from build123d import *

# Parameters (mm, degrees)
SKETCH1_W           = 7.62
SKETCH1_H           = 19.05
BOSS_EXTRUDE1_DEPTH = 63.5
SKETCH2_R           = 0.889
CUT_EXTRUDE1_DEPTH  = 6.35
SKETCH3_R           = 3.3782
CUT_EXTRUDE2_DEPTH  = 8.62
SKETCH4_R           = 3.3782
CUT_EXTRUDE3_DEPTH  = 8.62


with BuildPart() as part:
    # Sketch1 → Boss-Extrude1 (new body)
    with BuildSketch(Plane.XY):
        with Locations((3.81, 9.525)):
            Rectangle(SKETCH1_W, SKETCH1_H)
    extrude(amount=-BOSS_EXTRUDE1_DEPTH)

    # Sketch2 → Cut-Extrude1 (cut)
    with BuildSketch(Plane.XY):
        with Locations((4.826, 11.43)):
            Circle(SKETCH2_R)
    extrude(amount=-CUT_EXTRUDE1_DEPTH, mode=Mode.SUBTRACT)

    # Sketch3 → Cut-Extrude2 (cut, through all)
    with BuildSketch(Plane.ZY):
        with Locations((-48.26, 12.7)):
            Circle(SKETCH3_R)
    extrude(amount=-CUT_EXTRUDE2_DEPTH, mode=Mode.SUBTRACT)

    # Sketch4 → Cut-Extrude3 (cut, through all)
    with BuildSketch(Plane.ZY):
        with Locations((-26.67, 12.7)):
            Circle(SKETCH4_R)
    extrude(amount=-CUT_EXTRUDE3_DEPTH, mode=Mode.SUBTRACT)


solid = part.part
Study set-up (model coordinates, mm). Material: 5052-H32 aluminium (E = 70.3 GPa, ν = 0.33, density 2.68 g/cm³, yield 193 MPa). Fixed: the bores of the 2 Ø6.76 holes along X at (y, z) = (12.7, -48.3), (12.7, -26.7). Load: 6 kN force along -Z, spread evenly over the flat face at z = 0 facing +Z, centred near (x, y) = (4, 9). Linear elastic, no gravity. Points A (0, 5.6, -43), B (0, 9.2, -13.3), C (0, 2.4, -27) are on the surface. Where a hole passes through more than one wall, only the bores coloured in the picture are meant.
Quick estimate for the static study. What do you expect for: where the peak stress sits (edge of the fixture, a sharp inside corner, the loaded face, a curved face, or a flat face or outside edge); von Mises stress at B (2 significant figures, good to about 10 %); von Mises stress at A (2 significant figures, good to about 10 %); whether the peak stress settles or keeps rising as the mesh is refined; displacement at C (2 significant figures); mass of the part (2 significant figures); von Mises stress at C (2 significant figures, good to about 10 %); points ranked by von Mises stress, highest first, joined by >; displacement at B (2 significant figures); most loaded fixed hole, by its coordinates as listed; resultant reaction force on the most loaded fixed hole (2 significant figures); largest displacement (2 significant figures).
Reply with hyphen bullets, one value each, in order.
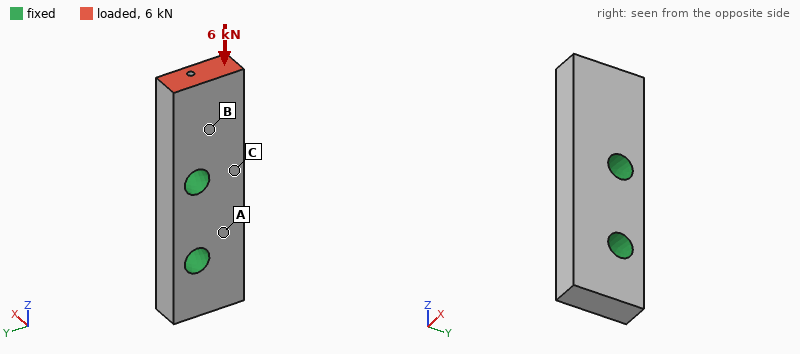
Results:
- edge of the fixture
- 45 MPa
- 12 MPa
- keeps rising
- 5.6 µm
- 23 g
- 30 MPa
- B > C > A
- 11 µm
- (12.7, -26.7)
- 5.2 kN
- 26 µm
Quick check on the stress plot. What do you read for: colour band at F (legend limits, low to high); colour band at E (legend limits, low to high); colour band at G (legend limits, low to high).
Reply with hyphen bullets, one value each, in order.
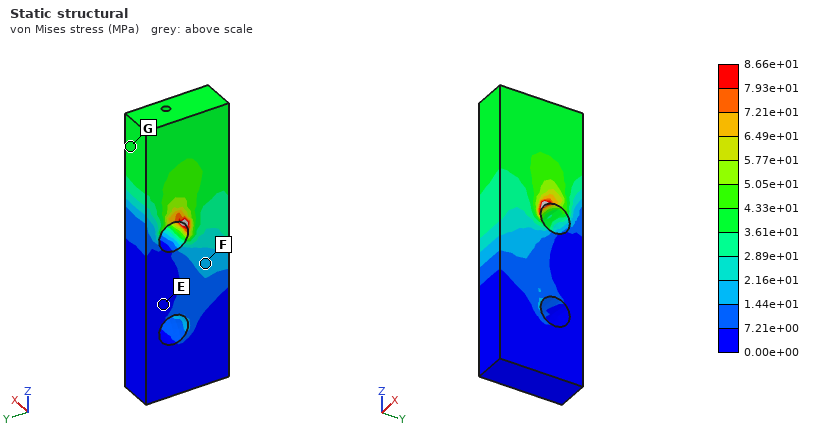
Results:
- 1.44e+01 to 2.16e+01 MPa
- 0.00e+00 to 7.21e+00 MPa
- 3.61e+01 to 4.33e+01 MPa
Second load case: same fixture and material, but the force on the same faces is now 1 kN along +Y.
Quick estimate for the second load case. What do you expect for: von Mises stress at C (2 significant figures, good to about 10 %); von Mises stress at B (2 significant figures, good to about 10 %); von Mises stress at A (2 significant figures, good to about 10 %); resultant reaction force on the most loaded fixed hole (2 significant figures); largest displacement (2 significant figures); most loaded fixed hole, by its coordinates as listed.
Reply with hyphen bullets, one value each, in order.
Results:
- 29 MPa
- 19 MPa
- 11 MPa
- 1.6 kN
- 41 µm
- (12.7, -26.7)
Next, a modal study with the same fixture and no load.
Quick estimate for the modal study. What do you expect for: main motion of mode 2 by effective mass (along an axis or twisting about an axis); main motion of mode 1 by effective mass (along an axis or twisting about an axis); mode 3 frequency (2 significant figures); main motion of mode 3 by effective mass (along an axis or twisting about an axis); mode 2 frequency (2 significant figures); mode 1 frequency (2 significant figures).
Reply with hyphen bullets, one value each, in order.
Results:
- along Y
- along X
- 20 kHz
- twisting about Z
- 15 kHz
- 9200 Hz
